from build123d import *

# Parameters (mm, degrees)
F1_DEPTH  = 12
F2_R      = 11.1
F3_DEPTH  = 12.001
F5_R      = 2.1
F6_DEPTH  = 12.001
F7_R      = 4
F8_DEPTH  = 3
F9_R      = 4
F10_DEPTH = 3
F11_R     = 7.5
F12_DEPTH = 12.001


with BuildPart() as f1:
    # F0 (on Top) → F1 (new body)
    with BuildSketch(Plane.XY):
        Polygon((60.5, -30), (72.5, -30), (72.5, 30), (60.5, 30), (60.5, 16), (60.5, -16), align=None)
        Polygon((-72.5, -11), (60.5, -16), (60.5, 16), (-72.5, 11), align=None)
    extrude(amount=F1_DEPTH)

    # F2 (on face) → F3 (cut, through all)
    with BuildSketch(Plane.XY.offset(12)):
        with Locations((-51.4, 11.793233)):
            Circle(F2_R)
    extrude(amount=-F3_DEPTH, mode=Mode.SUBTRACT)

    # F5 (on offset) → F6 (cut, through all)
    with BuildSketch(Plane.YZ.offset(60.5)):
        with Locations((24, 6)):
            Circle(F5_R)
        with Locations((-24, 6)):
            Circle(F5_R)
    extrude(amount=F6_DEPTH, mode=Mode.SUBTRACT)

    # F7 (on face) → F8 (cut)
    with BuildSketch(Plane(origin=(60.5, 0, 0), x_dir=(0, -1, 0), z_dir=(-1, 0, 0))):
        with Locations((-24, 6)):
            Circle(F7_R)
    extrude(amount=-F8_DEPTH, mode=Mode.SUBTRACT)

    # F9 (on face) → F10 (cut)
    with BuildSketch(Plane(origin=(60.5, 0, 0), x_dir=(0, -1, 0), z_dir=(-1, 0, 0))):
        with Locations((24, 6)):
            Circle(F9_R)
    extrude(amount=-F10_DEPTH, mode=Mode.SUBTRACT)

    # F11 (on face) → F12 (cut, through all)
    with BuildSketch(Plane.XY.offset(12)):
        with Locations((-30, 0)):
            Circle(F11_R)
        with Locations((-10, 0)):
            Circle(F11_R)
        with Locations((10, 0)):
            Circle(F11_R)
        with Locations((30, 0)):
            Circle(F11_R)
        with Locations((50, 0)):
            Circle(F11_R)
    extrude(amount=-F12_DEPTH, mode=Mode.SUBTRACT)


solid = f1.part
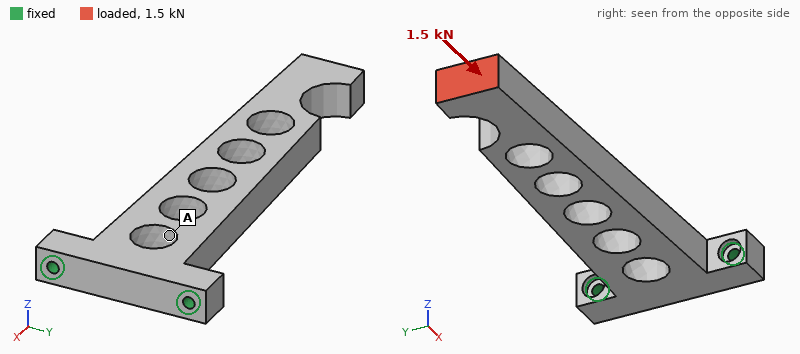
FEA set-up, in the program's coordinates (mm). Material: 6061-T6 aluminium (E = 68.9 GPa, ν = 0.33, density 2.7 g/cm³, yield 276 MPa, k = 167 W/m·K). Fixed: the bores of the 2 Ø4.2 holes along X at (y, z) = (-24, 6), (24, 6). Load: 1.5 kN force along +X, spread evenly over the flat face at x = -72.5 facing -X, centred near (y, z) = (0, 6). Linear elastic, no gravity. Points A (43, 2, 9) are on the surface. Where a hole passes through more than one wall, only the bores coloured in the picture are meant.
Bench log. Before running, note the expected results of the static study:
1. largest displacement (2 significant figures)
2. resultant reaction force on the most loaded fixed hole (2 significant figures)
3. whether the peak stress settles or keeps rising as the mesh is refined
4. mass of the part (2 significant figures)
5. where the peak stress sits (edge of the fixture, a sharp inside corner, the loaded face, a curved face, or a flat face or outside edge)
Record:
57 µm
830 N
keeps rising
100 g
edge of the fixture
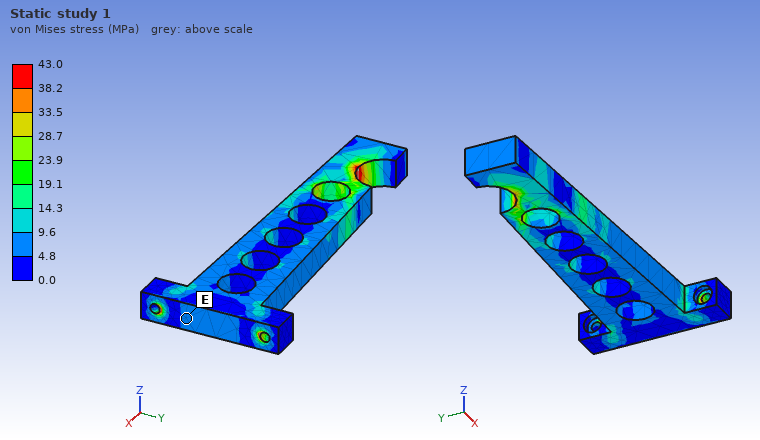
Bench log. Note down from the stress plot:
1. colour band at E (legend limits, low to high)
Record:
4.8 to 9.6 MPa
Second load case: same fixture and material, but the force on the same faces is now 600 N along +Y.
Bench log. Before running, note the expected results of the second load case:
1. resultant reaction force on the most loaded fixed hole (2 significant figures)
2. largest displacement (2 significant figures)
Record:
2.1 kN
0.47 mm
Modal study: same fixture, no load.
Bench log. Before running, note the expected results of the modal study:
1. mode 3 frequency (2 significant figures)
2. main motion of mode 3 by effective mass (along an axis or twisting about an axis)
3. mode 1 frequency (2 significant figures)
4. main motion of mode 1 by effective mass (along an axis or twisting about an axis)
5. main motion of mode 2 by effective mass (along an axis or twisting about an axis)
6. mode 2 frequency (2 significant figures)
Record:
2300 Hz
along Z
430 Hz
along Z
along Y
1300 Hz
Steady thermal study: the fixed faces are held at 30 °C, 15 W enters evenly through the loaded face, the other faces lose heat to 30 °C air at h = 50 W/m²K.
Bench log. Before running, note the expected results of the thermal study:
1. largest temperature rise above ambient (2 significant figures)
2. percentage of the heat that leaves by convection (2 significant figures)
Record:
43 K
61 %
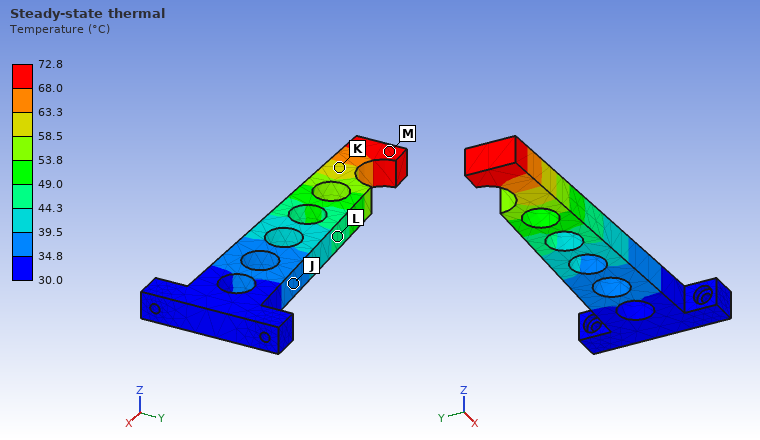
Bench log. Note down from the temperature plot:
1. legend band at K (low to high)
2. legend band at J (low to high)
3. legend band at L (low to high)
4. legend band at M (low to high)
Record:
58.5 to 63.3 °C
34.8 to 39.5 °C
44.3 to 49.0 °C
68.0 to 72.8 °C
